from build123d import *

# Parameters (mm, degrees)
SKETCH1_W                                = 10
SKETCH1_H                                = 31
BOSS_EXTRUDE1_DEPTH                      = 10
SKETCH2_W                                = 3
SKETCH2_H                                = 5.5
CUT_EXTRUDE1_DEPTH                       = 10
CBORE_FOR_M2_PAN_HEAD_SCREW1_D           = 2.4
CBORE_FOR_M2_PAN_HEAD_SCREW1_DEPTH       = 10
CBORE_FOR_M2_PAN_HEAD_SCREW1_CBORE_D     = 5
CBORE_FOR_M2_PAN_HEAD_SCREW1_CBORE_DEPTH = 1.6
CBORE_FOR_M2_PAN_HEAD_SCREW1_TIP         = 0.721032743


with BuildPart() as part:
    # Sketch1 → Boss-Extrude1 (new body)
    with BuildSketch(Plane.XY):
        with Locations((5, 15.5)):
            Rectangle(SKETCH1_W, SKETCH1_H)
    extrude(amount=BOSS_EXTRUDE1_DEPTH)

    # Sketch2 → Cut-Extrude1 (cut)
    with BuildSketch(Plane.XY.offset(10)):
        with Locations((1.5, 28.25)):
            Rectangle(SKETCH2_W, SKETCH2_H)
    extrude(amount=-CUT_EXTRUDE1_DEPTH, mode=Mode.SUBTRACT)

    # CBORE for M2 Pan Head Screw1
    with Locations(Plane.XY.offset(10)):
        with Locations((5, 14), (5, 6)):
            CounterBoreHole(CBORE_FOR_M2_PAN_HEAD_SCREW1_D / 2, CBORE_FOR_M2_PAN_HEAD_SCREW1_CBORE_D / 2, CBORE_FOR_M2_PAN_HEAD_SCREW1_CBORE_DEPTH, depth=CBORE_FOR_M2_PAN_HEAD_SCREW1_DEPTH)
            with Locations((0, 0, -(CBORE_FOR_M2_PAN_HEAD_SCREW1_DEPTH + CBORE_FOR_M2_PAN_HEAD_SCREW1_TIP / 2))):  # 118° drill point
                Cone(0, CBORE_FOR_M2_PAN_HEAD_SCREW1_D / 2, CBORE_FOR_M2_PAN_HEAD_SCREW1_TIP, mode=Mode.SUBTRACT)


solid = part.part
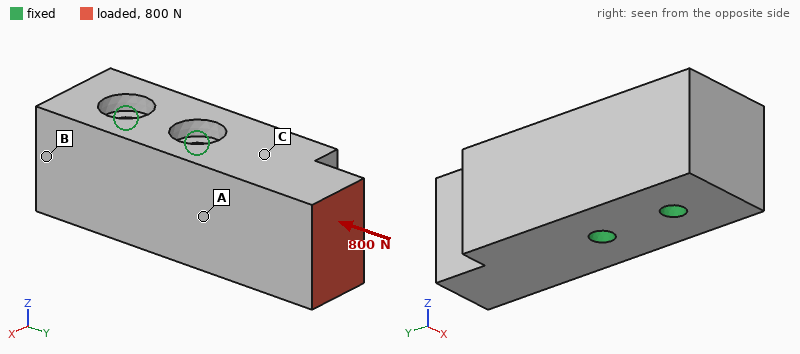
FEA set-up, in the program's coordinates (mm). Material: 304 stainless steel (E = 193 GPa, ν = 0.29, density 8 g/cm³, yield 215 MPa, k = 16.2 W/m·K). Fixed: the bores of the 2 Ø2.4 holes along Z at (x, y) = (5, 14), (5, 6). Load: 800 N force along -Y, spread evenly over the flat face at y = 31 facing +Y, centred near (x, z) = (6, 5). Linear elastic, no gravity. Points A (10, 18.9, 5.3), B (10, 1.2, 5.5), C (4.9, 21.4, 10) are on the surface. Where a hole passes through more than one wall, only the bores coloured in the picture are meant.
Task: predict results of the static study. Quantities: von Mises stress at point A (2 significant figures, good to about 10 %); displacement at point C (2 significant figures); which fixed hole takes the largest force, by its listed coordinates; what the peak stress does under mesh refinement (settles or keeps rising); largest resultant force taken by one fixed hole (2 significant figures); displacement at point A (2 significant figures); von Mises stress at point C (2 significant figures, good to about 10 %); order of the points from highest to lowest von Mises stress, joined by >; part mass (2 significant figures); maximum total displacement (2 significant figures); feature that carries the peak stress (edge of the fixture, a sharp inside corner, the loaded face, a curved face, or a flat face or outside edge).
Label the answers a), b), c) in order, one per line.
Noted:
a) 14 MPa
b) 0.64 µm
c) (5, 14)
d) keeps rising
e) 660 N
f) 0.71 µm
g) 8.7 MPa
h) A > C > B
i) 22 g
j) 2.1 µm
k) edge of the fixture
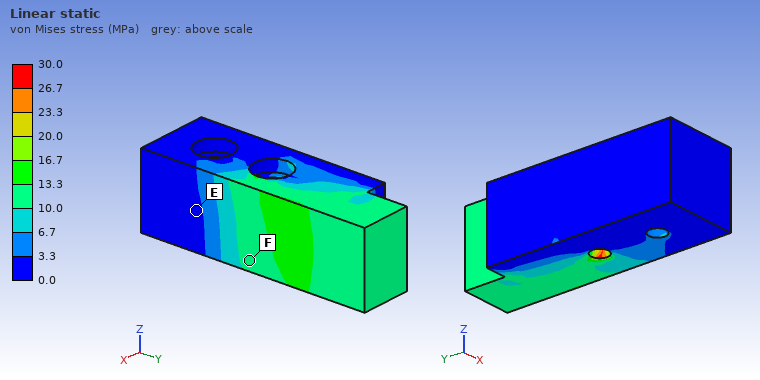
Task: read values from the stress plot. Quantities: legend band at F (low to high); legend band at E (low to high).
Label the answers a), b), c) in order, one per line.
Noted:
a) 10.0 to 13.3 MPa
b) 0.0 to 3.3 MPa
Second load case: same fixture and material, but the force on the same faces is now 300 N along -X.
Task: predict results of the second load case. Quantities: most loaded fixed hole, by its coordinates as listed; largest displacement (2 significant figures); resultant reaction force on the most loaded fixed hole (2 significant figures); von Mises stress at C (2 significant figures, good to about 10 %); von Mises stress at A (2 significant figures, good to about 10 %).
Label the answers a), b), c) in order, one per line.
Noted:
a) (5, 14)
b) 7.1 µm
c) 700 N
d) 8.2 MPa
e) 23 MPa
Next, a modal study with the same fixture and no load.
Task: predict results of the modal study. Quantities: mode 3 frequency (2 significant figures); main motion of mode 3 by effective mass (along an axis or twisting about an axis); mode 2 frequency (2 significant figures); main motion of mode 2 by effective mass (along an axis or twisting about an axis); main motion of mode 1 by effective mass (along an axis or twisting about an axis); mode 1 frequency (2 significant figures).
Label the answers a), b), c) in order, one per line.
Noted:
a) 43 kHz
b) twisting about Y
c) 21 kHz
d) along Z
e) along X
f) 19 kHz
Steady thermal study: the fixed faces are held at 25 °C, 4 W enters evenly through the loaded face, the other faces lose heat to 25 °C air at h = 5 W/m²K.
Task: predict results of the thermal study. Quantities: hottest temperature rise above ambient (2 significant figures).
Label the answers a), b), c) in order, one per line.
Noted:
a) 51 K
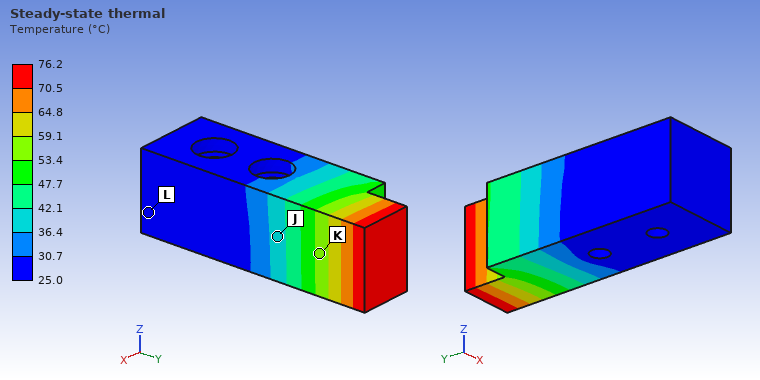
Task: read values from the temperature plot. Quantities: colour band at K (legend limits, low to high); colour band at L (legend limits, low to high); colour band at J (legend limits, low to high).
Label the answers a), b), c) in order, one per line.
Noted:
a) 53.4 to 59.1 °C
b) 25.0 to 30.7 °C
c) 36.4 to 42.1 °C
